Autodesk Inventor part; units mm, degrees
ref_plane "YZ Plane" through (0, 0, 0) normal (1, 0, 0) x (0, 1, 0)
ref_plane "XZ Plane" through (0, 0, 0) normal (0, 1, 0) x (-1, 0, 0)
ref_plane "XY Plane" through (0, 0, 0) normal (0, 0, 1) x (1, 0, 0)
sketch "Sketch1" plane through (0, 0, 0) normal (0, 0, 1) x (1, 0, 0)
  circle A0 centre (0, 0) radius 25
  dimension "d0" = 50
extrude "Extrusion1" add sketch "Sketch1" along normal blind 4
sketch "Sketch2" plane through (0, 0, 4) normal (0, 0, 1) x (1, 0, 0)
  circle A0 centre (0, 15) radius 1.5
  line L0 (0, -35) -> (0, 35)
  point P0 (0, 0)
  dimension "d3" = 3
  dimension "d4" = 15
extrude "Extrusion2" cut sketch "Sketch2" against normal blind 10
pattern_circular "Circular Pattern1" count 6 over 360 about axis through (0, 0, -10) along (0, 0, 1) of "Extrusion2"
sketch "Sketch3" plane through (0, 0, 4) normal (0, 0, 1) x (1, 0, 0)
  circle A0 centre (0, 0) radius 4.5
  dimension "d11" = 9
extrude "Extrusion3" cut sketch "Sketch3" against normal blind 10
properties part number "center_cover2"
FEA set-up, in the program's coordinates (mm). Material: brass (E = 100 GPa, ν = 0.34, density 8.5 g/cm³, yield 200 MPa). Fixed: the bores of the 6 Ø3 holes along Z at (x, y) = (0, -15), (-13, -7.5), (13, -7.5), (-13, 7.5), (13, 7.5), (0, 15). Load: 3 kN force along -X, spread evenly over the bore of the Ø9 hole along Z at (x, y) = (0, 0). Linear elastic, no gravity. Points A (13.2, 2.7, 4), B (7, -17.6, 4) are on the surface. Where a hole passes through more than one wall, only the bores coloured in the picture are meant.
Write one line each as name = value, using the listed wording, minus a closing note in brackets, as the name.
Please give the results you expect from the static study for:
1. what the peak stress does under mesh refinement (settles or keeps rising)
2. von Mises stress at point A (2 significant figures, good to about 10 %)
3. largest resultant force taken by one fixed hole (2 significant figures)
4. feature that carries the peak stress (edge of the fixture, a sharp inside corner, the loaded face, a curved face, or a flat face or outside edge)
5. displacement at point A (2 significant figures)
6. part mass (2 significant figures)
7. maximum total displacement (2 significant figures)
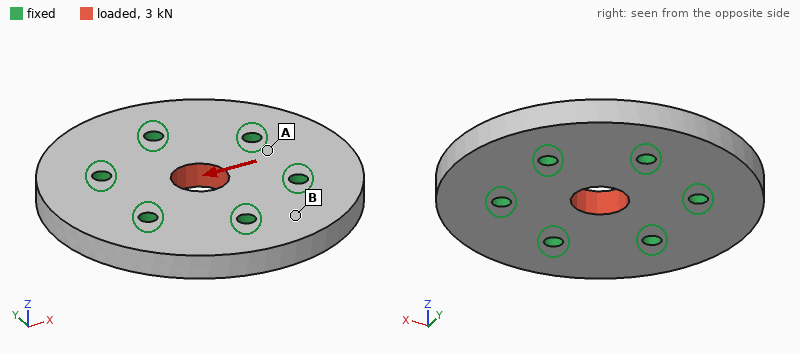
what the peak stress does under mesh refinement = keeps rising
von Mises stress at point A = 9.6 MPa
largest resultant force taken by one fixed hole = 680 N
feature that carries the peak stress = edge of the fixture
displacement at point A = 0.86 µm
part mass = 63 g
maximum total displacement = 2.6 µm
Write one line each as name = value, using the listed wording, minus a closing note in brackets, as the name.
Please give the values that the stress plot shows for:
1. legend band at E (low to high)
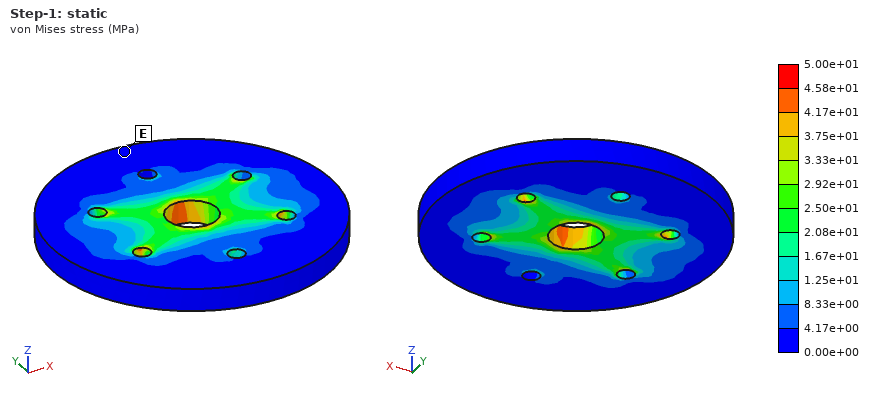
legend band at E = 0.00e+00 to 4.17e+00 MPa
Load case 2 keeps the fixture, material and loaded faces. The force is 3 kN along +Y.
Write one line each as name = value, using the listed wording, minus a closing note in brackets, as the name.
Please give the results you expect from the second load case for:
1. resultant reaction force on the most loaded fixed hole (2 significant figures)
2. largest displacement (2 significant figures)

resultant reaction force on the most loaded fixed hole = 770 N
largest displacement = 2.6 µm
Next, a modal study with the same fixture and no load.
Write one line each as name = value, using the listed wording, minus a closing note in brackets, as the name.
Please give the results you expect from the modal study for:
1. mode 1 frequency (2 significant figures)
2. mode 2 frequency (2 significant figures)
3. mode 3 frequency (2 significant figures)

mode 1 frequency = 17 kHz
mode 2 frequency = 17 kHz
mode 3 frequency = 17 kHz
